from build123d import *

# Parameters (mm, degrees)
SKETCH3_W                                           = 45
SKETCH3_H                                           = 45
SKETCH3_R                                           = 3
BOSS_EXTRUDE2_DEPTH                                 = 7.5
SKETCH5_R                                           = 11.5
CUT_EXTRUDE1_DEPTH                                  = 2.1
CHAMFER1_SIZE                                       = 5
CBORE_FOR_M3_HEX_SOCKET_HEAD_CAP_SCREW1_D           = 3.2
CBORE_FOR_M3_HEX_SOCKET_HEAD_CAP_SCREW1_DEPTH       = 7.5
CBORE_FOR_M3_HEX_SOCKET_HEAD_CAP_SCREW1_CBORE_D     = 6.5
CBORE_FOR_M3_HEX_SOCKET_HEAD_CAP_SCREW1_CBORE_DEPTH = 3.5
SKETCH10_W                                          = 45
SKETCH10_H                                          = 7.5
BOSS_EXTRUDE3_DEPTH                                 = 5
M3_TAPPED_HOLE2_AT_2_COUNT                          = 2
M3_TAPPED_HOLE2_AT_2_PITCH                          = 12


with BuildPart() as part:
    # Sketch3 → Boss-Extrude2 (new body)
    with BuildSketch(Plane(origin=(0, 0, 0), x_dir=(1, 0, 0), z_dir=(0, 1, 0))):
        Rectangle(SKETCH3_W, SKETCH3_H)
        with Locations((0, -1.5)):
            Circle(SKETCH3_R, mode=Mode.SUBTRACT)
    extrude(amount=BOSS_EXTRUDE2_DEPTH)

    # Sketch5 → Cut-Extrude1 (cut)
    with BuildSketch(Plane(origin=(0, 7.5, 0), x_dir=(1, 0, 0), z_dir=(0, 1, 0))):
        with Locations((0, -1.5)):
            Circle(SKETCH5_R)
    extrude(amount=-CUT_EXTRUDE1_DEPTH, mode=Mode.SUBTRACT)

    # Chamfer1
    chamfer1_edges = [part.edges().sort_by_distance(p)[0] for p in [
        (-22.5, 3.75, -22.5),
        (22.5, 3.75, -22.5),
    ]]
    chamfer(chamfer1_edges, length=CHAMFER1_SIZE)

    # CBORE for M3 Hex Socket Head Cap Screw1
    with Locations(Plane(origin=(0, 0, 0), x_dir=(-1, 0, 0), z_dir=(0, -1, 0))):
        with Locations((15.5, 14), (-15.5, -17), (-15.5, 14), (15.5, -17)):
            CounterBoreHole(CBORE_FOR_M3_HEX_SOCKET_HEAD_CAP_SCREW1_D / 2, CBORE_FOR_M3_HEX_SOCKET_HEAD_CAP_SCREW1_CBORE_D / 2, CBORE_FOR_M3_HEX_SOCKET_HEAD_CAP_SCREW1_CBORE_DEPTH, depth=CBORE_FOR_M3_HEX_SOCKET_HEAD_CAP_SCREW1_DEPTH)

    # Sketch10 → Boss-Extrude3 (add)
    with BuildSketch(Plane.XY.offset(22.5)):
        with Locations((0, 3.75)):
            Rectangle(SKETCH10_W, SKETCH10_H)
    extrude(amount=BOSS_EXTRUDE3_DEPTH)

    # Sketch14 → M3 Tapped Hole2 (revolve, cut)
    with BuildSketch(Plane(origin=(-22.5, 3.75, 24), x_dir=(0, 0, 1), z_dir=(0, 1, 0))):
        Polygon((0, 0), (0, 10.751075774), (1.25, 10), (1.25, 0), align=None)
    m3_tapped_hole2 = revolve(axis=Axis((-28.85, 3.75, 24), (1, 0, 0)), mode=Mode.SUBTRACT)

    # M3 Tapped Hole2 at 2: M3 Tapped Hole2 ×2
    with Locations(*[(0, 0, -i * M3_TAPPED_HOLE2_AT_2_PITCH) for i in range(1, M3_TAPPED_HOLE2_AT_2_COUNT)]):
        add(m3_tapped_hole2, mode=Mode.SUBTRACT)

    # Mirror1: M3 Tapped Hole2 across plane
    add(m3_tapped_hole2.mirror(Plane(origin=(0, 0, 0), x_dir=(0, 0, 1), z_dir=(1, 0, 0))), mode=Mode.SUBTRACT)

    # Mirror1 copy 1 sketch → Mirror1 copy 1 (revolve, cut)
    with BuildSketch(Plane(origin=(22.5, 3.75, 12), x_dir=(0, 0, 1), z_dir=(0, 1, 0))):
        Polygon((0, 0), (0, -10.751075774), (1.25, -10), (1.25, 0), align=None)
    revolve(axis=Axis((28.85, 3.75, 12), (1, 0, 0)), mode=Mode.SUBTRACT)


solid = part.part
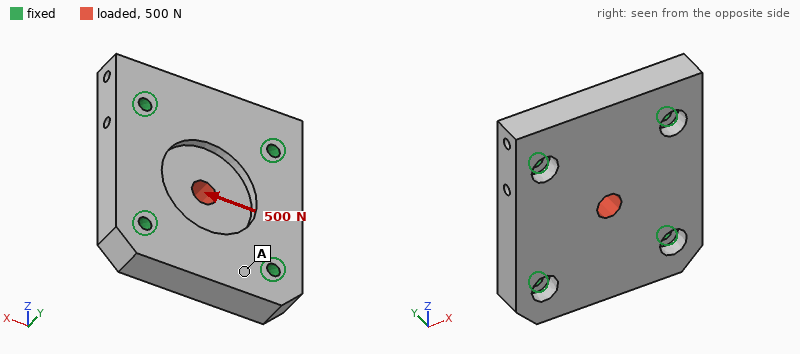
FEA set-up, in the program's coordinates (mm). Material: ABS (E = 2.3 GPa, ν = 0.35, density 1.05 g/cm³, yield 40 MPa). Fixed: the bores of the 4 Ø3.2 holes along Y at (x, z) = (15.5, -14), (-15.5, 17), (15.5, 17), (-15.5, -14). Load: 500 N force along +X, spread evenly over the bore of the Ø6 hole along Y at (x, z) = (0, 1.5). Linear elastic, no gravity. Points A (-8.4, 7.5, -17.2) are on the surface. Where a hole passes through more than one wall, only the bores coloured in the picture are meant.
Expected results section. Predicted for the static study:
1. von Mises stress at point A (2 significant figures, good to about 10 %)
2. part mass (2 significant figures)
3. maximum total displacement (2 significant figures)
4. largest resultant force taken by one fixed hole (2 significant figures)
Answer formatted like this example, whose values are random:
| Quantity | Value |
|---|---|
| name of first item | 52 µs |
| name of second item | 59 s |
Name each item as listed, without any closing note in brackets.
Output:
| Quantity | Value |
|---|---|
| von Mises stress at point A | 0.89 MPa |
| part mass | 16 g |
| maximum total displacement | 32 µm |
| largest resultant force taken by one fixed hole | 140 N |
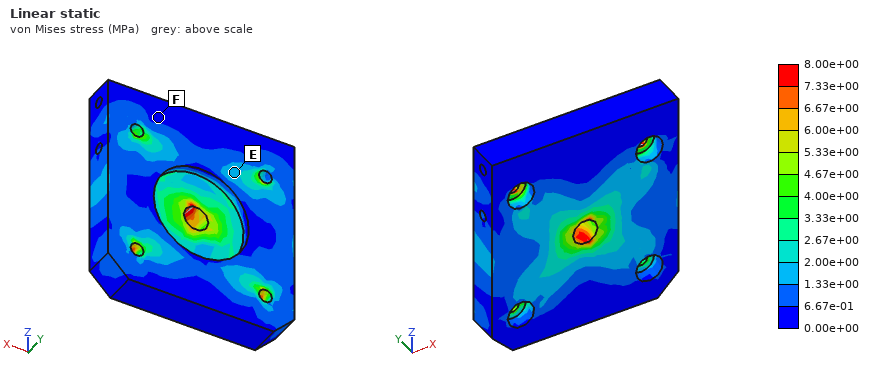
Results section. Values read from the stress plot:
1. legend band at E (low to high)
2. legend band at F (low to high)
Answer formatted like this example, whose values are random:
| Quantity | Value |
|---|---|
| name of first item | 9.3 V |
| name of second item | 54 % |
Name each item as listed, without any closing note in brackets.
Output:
| Quantity | Value |
|---|---|
| legend band at E | 1.33e+00 to 2.00e+00 MPa |
| legend band at F | 0.00e+00 to 6.67e-01 MPa |
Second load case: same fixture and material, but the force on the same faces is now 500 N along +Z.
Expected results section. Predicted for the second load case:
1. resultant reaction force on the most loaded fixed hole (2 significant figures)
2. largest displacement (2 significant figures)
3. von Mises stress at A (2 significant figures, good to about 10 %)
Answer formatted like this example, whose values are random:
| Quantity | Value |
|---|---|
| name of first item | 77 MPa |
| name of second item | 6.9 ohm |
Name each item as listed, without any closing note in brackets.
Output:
| Quantity | Value |
|---|---|
| resultant reaction force on the most loaded fixed hole | 140 N |
| largest displacement | 31 µm |
| von Mises stress at A | 1.1 MPa |
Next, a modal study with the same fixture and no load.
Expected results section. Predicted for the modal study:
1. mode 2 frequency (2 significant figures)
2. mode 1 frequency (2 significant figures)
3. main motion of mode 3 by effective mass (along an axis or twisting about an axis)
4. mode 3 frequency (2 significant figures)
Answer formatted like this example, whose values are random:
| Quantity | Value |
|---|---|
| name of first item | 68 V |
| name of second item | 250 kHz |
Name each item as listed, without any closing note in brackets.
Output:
| Quantity | Value |
|---|---|
| mode 2 frequency | 5600 Hz |
| mode 1 frequency | 5500 Hz |
| main motion of mode 3 by effective mass | twisting about X |
| mode 3 frequency | 6400 Hz |
